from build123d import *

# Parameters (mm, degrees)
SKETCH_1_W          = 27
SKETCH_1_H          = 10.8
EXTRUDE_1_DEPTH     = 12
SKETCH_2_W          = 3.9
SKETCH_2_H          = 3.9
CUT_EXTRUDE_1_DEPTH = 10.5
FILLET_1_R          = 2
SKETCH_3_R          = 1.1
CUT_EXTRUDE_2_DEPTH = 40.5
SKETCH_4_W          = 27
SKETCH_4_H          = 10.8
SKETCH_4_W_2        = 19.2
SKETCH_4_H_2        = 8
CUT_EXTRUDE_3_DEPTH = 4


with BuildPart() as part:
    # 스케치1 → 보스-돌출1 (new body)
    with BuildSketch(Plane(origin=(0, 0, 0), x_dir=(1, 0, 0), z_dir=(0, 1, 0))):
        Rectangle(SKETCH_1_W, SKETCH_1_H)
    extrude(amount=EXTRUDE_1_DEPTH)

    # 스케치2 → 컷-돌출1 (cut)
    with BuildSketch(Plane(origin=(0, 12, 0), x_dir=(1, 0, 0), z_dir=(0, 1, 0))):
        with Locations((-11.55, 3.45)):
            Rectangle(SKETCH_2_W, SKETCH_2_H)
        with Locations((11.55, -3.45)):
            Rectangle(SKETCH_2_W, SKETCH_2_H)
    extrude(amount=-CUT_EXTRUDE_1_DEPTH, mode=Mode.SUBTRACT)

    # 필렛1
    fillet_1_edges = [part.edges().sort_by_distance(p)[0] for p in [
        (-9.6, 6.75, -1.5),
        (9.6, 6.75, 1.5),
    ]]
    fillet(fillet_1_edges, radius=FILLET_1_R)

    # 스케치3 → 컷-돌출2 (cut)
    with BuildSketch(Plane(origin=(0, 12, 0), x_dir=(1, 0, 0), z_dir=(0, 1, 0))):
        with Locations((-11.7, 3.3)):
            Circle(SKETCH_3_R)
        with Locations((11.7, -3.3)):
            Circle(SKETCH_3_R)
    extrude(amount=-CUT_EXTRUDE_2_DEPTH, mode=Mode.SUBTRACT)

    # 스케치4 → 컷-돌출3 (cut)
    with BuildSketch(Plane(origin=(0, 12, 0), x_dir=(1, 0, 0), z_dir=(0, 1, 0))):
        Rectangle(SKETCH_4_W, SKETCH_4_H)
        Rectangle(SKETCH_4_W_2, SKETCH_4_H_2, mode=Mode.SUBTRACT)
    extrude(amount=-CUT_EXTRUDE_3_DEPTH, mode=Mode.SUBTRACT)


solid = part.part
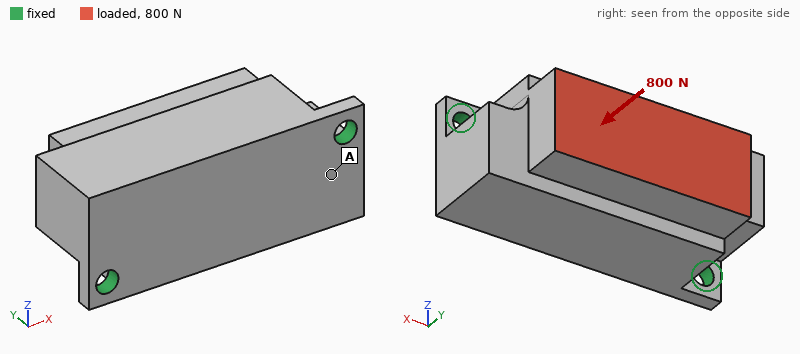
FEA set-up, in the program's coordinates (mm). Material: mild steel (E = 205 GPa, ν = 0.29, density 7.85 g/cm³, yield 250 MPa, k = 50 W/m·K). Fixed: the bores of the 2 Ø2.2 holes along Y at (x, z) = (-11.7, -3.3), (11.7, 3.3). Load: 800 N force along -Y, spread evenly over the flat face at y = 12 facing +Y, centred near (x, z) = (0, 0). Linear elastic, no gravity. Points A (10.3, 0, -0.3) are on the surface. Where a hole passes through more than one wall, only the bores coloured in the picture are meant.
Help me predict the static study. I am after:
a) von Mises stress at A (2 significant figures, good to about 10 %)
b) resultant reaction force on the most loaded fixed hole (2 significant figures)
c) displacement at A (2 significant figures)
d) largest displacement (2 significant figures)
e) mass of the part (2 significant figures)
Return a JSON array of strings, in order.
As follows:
["18 MPa", "440 N", "1.7 µm", "2.5 µm", "22 g"]
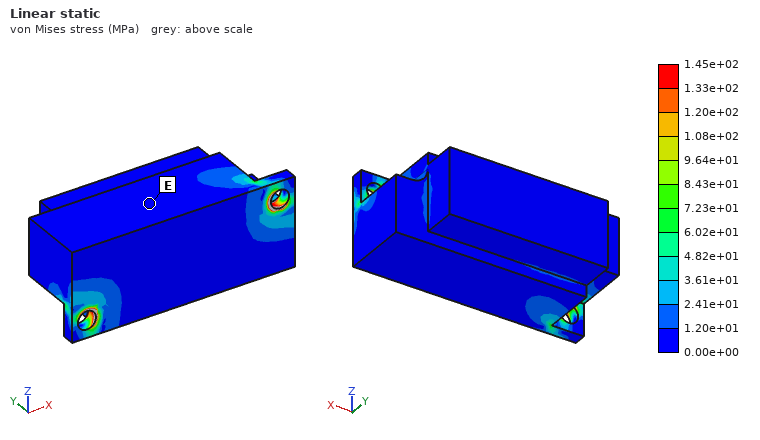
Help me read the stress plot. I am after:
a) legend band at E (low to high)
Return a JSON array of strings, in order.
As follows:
["0.00e+00 to 1.20e+01 MPa"]
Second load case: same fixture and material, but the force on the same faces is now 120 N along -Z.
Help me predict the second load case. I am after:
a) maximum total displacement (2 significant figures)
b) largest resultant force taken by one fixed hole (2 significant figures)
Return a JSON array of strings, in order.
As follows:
["17 µm", "67 N"]
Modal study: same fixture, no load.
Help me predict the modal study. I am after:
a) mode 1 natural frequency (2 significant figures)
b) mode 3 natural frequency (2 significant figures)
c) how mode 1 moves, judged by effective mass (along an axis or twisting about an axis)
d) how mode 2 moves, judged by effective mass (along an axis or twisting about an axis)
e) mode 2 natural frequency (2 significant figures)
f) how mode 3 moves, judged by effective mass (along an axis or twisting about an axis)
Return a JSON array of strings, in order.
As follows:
["5200 Hz", "27 kHz", "along Z", "along Y", "21 kHz", "along X"]
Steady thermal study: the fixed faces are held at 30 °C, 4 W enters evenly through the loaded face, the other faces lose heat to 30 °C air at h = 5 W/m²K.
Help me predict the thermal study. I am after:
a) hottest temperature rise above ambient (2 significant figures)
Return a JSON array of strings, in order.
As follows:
["15 K"]
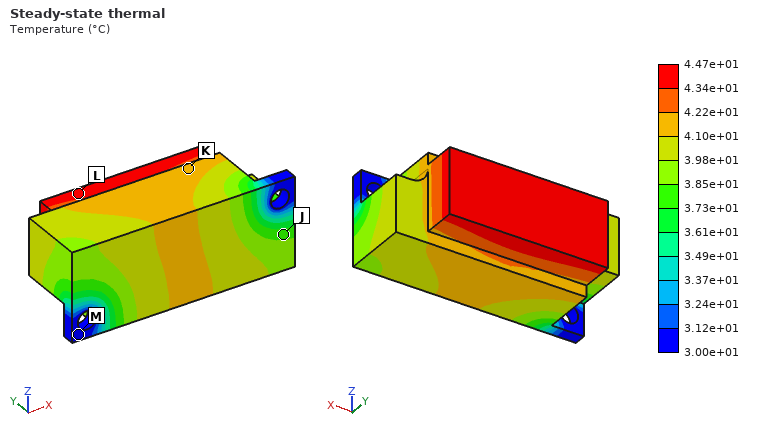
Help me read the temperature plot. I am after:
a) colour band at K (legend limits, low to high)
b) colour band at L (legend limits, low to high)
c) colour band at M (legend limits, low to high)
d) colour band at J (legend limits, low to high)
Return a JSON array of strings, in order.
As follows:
["4.10e+01 to 4.22e+01 °C", "4.34e+01 to 4.47e+01 °C", "3.00e+01 to 3.12e+01 °C", "3.73e+01 to 3.85e+01 °C"]
